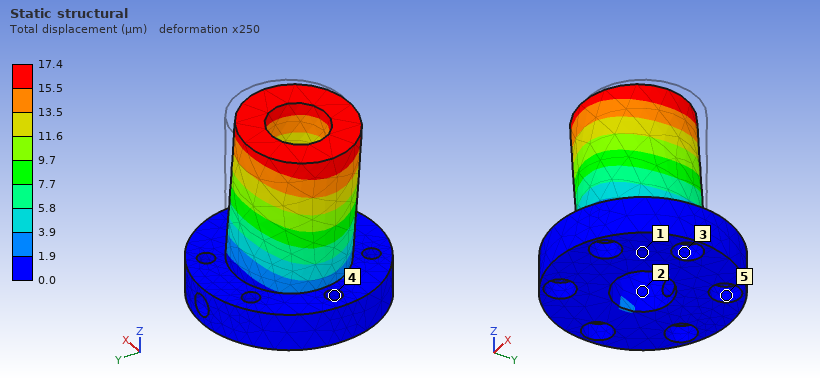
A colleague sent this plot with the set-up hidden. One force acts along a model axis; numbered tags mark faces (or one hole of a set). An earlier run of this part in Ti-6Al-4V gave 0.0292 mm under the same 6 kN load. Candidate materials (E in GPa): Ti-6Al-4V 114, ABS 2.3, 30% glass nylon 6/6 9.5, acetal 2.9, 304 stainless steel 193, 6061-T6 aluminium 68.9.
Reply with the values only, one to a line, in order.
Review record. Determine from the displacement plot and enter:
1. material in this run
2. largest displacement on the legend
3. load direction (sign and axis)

304 stainless steel
17.4 µm
-X
